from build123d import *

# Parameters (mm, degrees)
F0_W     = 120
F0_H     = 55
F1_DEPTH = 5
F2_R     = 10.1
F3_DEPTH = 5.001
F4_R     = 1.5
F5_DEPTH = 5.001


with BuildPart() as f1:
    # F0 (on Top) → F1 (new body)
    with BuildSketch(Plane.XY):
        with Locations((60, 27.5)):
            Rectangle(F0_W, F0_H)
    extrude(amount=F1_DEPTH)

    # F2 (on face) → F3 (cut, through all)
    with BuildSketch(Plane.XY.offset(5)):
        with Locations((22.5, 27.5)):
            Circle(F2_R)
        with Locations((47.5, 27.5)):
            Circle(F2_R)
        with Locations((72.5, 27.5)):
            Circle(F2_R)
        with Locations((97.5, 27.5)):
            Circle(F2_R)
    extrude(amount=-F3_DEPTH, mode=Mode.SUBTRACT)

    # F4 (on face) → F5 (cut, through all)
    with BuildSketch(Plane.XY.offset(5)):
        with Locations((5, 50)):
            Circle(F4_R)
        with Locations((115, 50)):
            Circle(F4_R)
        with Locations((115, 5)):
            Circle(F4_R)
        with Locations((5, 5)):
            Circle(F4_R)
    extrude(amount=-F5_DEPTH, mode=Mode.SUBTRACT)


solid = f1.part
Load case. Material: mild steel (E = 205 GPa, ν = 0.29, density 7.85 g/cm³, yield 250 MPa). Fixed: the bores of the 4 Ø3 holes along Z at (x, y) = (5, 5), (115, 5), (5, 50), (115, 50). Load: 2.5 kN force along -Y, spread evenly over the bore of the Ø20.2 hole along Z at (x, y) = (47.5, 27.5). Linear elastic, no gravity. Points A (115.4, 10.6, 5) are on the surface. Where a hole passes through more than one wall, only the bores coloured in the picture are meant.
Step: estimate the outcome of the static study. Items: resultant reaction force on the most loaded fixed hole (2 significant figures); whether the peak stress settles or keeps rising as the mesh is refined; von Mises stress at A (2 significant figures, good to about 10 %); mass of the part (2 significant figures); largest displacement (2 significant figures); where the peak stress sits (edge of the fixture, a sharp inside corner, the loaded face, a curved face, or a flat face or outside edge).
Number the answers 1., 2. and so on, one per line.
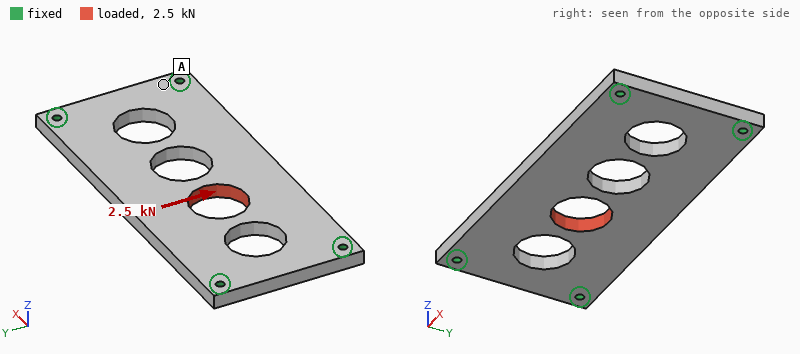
1. 1.1 kN
2. keeps rising
3. 8.5 MPa
4. 210 g
5. 11 µm
6. edge of the fixture
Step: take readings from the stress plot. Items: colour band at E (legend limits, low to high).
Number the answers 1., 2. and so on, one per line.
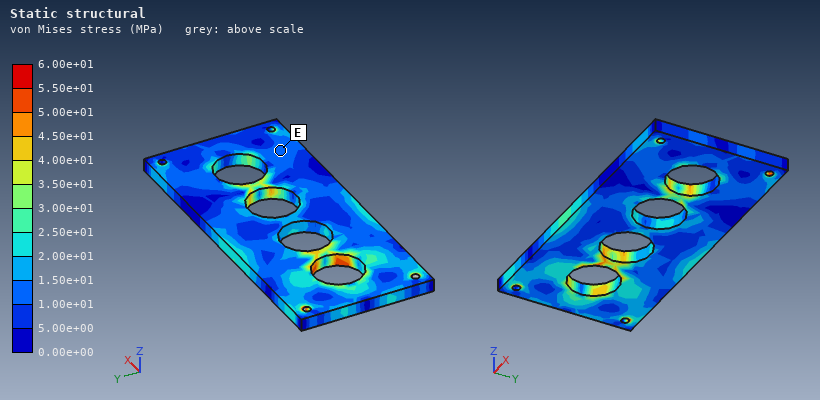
1. 1.00e+01 to 1.50e+01 MPa
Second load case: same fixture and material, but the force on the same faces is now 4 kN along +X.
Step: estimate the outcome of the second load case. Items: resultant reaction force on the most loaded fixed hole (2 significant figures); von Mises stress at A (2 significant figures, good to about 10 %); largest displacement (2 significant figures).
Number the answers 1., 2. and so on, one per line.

1. 1.2 kN
2. 5.1 MPa
3. 5.3 µm
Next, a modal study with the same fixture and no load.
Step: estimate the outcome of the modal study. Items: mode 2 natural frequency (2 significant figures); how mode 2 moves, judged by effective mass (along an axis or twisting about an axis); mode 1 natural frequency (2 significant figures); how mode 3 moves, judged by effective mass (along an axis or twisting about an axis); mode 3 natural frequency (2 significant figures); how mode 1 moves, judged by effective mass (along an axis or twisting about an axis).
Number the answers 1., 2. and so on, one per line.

1. 3100 Hz
2. twisting about X
3. 1900 Hz
4. twisting about Y
5. 5100 Hz
6. along Z
